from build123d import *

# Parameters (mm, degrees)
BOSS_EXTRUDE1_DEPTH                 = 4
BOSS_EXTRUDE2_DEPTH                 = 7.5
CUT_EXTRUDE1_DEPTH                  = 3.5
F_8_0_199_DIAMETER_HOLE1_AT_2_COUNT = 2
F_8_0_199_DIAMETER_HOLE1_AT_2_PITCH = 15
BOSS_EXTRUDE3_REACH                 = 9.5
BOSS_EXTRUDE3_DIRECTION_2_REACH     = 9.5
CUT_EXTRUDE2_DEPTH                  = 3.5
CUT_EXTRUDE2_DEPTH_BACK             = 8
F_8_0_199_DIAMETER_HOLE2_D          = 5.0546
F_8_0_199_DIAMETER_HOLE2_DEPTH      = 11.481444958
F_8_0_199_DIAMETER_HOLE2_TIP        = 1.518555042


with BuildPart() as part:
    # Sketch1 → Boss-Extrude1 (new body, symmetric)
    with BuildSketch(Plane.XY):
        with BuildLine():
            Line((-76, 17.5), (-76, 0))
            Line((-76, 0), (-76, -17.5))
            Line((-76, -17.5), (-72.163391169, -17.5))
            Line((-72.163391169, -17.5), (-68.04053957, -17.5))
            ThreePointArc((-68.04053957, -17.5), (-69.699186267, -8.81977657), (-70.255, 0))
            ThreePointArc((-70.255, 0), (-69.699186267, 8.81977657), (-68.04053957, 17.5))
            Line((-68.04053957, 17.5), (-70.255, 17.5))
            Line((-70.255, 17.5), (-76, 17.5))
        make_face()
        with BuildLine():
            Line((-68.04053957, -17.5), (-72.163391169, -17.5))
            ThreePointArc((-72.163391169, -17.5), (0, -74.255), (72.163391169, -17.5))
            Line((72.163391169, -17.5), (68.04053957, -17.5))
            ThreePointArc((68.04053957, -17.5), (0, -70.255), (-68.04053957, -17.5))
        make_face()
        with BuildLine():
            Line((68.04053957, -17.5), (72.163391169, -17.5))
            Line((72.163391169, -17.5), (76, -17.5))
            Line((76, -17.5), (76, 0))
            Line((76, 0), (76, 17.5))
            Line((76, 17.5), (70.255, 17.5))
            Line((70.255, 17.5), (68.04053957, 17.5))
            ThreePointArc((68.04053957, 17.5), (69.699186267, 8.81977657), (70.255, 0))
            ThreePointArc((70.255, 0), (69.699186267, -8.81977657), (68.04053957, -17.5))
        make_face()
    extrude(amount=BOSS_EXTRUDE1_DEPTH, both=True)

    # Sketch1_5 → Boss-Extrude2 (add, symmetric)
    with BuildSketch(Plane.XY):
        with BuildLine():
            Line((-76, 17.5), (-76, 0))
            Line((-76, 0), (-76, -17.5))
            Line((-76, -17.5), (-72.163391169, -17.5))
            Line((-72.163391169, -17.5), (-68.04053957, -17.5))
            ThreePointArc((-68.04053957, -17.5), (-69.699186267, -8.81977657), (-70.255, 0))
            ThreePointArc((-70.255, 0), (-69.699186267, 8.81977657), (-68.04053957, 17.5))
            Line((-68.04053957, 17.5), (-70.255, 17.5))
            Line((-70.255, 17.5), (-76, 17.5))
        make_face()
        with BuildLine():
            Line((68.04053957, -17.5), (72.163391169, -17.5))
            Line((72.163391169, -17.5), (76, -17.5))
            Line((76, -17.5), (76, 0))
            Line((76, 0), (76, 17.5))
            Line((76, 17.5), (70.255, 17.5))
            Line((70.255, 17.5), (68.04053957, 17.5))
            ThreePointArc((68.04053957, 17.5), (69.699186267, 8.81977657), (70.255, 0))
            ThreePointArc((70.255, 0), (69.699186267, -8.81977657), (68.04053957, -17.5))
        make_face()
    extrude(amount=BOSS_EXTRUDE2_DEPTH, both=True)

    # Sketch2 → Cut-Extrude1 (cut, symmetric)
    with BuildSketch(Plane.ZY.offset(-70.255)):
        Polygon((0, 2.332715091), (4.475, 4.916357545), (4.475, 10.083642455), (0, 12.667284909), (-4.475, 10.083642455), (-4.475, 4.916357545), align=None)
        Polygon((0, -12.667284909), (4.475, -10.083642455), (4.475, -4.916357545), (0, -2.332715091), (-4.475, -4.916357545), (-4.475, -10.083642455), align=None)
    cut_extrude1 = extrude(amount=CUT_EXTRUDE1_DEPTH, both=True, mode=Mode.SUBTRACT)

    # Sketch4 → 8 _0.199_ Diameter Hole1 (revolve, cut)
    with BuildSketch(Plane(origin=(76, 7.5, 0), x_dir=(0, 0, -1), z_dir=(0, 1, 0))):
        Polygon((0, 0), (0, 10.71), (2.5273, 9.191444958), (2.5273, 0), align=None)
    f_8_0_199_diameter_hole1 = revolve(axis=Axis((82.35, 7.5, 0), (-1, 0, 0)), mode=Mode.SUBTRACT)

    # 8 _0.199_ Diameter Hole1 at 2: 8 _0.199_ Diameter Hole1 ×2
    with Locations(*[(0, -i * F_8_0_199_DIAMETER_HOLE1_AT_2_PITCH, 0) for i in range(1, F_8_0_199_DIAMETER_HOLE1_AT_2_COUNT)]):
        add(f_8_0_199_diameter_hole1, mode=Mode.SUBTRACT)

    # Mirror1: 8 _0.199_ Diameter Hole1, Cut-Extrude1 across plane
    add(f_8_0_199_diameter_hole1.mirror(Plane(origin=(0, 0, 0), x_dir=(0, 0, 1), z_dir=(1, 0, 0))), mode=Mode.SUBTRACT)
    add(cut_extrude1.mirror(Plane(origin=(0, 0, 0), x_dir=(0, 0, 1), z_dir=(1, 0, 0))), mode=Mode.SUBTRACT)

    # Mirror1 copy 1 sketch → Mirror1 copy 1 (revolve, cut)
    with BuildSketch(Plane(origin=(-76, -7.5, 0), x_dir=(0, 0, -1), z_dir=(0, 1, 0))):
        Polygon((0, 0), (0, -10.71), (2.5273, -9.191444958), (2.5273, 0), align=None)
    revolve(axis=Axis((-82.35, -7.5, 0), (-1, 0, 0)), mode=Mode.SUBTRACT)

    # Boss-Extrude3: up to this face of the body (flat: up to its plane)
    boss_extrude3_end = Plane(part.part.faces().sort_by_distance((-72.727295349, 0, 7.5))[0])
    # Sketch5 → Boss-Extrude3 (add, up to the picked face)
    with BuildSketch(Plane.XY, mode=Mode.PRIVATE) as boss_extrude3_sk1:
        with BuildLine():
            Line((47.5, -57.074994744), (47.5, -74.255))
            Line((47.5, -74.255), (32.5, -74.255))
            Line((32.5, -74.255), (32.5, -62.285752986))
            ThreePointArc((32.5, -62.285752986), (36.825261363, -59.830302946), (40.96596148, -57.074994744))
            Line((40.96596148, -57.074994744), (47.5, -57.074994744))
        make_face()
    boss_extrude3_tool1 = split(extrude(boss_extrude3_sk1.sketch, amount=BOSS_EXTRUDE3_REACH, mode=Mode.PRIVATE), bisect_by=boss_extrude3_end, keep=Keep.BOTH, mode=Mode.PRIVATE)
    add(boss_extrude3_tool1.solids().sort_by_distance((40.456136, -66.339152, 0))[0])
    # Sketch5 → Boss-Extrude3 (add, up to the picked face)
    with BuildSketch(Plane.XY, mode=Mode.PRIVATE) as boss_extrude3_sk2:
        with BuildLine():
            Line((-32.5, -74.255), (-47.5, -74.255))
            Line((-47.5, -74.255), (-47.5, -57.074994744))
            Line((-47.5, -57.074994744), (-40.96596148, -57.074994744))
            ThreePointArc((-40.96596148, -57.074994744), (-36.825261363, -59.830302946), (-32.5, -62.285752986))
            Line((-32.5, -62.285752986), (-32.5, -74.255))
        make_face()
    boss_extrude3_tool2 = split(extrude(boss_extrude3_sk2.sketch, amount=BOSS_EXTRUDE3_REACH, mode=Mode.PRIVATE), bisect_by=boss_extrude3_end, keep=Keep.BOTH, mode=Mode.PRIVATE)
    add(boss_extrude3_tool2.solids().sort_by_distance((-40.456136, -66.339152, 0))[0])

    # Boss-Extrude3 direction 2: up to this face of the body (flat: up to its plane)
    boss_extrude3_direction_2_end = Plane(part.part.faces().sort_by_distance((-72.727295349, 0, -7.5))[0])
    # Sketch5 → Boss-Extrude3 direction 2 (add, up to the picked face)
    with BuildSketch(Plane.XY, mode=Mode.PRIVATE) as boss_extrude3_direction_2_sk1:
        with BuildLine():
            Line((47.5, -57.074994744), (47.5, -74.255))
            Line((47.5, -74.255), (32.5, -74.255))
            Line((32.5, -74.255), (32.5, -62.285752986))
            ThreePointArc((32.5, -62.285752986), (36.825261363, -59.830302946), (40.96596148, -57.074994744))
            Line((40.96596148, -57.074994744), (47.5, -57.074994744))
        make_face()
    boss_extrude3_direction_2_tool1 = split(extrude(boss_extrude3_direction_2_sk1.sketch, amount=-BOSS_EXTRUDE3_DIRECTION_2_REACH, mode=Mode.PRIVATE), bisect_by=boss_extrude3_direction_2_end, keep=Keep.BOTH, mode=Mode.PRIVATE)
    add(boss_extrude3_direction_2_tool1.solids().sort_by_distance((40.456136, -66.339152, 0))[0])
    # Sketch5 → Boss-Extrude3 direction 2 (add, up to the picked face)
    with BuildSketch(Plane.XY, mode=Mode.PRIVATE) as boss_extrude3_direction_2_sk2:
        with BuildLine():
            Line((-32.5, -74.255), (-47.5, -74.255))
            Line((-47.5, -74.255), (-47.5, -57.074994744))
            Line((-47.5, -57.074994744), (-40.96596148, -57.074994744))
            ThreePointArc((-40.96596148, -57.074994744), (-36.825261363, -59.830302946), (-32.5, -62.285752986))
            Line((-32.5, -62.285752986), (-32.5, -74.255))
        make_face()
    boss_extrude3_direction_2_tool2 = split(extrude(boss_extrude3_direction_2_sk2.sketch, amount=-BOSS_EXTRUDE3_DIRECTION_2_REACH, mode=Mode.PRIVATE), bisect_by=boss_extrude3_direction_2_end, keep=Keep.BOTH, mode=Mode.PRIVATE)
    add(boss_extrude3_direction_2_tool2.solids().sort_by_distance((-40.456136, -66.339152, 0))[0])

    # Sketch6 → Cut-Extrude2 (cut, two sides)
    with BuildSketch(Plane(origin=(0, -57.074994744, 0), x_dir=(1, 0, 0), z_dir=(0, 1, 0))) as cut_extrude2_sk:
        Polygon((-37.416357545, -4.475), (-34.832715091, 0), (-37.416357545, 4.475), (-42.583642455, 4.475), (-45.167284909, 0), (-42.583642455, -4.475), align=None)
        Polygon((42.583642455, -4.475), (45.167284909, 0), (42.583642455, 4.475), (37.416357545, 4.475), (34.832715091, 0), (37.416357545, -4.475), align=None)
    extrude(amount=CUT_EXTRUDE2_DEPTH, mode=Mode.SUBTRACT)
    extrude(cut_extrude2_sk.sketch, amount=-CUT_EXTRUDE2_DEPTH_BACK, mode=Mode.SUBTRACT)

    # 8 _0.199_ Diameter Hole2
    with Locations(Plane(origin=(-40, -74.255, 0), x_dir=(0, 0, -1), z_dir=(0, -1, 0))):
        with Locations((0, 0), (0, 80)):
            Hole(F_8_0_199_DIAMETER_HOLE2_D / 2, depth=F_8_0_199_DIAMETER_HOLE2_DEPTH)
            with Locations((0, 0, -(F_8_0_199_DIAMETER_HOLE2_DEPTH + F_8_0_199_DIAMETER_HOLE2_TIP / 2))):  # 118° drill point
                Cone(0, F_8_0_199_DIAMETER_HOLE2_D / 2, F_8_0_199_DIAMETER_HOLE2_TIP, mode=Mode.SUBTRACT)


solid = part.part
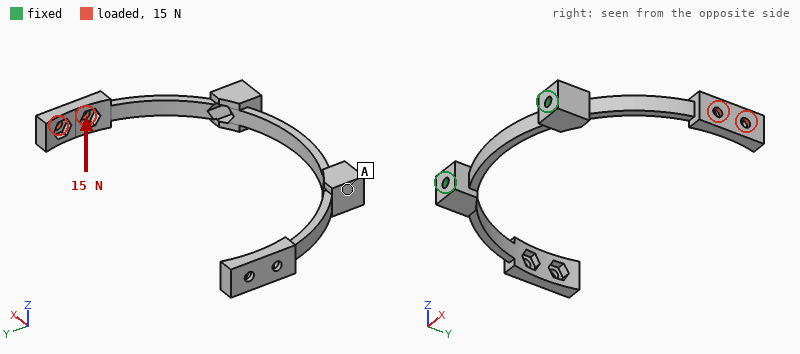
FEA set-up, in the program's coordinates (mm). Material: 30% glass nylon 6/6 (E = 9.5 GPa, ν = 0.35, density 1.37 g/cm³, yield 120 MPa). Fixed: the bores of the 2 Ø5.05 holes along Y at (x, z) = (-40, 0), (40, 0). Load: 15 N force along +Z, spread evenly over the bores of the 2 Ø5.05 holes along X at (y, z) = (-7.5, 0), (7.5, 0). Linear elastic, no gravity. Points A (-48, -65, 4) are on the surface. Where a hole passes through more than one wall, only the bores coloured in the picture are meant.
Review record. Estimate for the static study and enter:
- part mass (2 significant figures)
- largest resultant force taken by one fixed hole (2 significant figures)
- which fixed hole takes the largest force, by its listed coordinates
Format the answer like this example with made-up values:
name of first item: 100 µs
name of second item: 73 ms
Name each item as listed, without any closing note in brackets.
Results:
part mass: 22 g
largest resultant force taken by one fixed hole: 16 N
which fixed hole takes the largest force, by its listed coordinates: (40, 0)
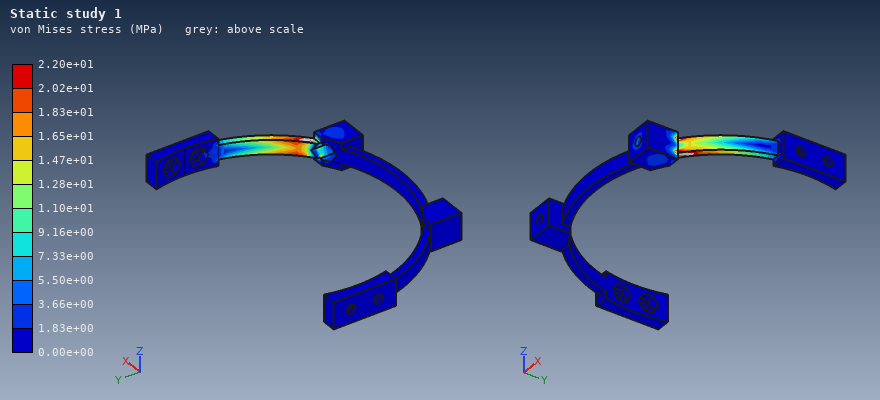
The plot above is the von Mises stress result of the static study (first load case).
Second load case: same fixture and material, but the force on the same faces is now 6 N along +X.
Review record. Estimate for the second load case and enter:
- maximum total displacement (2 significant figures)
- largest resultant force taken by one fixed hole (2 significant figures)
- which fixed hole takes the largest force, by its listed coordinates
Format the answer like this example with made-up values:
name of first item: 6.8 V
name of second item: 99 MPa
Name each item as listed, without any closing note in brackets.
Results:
maximum total displacement: 2.0 mm
largest resultant force taken by one fixed hole: 6.0 N
which fixed hole takes the largest force, by its listed coordinates: (40, 0)
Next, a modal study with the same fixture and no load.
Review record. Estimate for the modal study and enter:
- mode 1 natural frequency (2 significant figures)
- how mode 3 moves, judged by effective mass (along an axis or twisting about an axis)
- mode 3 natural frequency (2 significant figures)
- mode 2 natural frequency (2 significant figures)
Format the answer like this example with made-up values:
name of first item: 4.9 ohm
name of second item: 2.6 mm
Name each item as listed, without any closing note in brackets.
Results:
mode 1 natural frequency: 150 Hz
how mode 3 moves, judged by effective mass: along Z
mode 3 natural frequency: 280 Hz
mode 2 natural frequency: 150 Hz
